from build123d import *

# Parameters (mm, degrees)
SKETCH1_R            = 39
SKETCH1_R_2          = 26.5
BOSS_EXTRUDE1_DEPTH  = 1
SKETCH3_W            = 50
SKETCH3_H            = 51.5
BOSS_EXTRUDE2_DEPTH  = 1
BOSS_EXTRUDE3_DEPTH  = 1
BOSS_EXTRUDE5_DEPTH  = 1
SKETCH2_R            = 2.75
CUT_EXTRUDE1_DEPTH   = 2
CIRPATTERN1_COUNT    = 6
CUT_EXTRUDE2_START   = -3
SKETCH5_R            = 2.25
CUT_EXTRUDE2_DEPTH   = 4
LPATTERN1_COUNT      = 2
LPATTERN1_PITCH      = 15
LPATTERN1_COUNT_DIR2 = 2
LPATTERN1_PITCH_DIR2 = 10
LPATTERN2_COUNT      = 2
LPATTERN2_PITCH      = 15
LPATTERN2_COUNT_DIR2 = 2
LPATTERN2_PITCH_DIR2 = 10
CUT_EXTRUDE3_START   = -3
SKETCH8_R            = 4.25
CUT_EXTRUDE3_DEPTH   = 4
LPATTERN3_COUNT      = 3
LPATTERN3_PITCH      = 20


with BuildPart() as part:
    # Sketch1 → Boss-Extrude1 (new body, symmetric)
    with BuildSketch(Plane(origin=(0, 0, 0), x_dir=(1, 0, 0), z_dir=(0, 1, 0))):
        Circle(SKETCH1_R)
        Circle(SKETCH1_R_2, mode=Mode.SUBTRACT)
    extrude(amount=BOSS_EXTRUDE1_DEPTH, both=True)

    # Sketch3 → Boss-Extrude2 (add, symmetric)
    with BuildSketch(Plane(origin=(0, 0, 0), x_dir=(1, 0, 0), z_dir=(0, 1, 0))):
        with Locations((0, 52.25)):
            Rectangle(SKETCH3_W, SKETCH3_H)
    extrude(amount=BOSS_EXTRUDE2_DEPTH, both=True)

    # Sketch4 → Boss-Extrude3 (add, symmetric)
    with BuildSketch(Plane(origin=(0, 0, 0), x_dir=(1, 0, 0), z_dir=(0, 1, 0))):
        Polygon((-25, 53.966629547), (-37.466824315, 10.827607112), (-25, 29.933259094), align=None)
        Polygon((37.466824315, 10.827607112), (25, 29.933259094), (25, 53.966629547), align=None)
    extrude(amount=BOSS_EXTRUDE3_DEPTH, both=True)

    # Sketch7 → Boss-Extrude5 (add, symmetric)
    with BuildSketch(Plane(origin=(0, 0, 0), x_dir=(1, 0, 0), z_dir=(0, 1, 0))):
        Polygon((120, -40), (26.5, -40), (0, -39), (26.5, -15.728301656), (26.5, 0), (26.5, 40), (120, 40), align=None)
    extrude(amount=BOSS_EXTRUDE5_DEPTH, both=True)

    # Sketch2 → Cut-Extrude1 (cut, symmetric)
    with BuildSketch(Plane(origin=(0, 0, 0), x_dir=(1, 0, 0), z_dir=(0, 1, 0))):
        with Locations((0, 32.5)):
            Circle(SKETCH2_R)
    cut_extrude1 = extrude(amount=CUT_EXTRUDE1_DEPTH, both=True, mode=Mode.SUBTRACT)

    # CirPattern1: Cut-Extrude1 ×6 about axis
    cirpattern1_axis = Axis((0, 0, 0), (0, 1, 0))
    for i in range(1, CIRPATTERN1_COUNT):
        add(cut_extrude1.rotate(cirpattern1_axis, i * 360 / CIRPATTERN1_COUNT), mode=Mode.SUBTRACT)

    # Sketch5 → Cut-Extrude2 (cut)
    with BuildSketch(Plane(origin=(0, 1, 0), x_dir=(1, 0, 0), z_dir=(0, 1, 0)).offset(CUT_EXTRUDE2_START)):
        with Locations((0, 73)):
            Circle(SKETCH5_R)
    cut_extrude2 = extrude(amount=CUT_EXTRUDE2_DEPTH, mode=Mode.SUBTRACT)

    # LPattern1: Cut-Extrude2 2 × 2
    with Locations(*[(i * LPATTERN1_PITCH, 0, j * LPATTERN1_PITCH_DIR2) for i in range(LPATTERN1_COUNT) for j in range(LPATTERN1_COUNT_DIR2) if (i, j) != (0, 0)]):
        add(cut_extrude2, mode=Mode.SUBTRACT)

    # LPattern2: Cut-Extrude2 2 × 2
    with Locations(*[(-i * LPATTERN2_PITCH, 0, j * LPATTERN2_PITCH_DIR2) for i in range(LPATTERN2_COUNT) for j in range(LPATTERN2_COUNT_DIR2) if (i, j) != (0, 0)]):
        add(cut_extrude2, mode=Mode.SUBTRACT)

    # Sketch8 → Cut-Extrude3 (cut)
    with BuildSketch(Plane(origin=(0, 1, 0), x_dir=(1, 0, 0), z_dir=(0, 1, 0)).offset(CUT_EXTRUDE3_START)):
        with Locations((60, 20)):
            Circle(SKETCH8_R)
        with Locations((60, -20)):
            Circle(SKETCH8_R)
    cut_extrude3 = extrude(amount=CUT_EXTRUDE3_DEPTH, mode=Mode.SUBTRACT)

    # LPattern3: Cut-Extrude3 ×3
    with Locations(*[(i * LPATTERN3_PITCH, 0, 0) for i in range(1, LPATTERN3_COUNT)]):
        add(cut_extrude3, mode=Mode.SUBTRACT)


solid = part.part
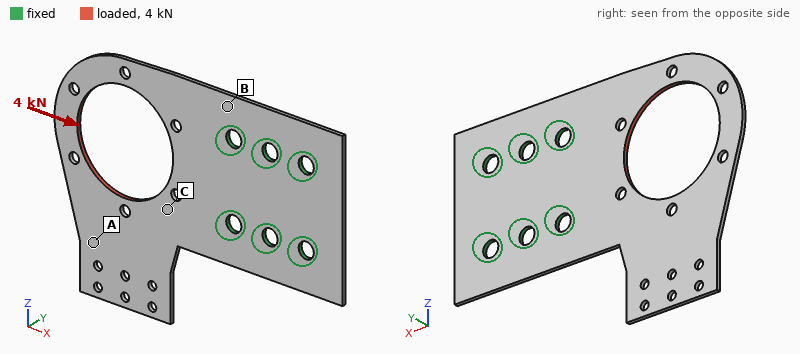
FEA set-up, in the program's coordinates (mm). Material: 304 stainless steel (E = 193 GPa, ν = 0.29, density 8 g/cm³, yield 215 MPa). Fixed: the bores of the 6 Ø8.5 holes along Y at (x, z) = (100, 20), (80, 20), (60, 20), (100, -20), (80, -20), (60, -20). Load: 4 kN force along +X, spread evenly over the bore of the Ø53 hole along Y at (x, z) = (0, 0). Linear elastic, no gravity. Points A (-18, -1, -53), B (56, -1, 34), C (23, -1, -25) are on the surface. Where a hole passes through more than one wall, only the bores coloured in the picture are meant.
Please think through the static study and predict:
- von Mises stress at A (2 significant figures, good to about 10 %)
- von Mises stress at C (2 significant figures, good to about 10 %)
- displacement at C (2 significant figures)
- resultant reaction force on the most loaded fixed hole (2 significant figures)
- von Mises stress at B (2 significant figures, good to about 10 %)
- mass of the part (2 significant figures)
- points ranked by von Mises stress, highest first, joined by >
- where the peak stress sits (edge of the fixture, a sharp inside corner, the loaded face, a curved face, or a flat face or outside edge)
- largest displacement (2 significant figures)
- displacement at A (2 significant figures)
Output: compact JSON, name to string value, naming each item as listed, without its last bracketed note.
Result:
{"von Mises stress at A": "11 MPa", "von Mises stress at C": "46 MPa", "displacement at C": "8.6 µm", "resultant reaction force on the most loaded fixed hole": "1.5 kN", "von Mises stress at B": "28 MPa", "mass of the part": "180 g", "points ranked by von Mises stress, highest first, joined by >": "C > B > A", "where the peak stress sits": "a curved face", "largest displacement": "40 µm", "displacement at A": "13 µm"}
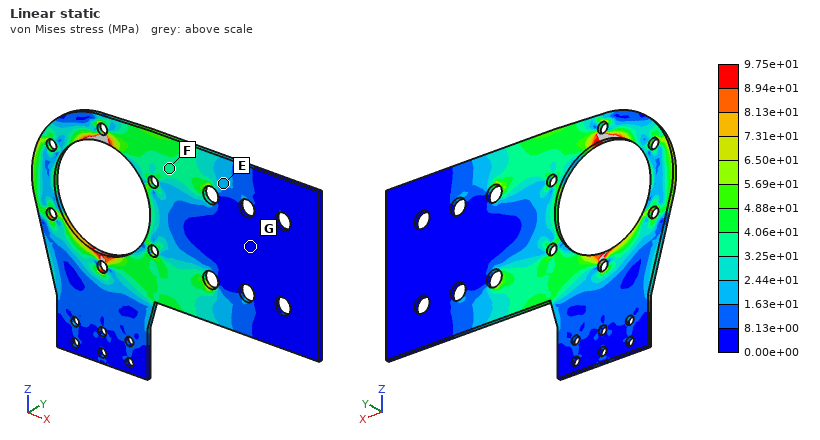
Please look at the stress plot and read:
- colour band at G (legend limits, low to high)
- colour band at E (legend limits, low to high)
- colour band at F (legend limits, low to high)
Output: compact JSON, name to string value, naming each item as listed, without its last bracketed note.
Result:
{"colour band at G": "0.00e+00 to 8.13e+00 MPa", "colour band at E": "1.63e+01 to 2.44e+01 MPa", "colour band at F": "3.25e+01 to 4.06e+01 MPa"}
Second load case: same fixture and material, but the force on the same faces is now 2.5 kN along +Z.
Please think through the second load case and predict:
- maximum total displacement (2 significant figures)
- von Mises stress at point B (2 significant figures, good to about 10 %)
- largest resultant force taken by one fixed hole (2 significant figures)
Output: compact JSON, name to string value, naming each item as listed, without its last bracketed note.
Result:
{"maximum total displacement": "0.15 mm", "von Mises stress at point B": "49 MPa", "largest resultant force taken by one fixed hole": "2.5 kN"}
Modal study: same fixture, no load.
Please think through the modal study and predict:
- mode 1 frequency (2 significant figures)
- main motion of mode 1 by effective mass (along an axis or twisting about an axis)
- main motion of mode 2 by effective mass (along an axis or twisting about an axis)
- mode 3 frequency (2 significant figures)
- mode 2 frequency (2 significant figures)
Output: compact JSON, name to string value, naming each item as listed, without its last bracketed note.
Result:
{"mode 1 frequency": "160 Hz", "main motion of mode 1 by effective mass": "along Y", "main motion of mode 2 by effective mass": "twisting about X", "mode 3 frequency": "720 Hz", "mode 2 frequency": "310 Hz"}
